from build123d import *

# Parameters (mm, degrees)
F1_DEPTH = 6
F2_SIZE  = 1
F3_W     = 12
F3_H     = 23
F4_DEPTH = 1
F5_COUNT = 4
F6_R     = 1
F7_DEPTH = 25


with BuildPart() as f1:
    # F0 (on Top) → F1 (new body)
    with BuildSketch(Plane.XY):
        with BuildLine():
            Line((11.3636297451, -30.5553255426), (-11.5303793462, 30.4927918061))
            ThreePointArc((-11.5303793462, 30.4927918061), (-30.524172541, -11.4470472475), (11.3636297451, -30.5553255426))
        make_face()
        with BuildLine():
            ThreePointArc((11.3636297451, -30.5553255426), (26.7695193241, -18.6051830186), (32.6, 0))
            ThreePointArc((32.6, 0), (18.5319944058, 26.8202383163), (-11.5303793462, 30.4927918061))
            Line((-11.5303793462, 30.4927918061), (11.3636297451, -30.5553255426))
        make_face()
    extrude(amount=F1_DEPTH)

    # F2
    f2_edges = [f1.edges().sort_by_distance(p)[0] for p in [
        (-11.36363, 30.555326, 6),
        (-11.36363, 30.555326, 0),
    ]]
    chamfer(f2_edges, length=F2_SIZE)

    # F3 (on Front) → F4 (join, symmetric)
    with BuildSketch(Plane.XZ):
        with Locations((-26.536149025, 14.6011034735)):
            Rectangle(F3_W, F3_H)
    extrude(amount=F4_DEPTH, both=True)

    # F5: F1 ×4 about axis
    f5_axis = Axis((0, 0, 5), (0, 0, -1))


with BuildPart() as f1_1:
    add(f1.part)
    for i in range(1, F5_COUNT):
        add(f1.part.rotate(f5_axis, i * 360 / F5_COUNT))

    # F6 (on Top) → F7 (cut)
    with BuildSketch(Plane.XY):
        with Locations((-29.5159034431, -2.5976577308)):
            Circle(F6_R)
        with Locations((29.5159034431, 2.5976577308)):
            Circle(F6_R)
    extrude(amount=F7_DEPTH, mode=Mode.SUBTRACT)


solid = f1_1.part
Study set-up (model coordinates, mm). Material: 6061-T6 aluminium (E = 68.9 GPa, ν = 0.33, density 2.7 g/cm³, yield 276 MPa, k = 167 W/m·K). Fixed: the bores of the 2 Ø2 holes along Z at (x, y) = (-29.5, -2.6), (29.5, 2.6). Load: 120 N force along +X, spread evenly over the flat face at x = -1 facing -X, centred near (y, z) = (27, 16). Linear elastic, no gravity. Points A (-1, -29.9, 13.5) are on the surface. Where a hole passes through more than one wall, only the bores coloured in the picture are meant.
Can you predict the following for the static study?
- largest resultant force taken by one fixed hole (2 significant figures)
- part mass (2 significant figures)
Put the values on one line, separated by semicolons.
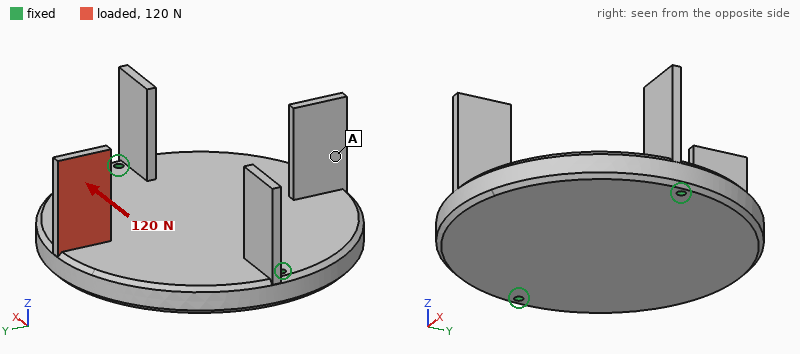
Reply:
90 N; 59 g
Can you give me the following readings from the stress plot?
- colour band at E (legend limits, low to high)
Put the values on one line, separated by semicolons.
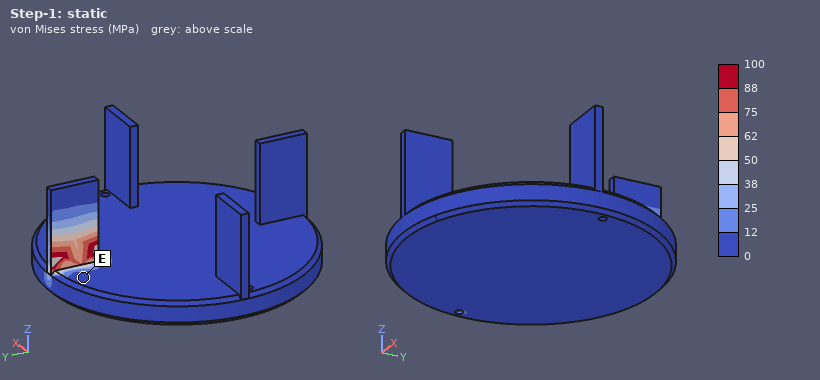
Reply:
0 to 12 MPa
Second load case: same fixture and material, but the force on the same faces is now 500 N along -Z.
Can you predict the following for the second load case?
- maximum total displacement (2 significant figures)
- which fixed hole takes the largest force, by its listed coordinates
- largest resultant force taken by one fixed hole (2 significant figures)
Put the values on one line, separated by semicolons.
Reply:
0.26 mm; (29.5, 2.6); 260 N
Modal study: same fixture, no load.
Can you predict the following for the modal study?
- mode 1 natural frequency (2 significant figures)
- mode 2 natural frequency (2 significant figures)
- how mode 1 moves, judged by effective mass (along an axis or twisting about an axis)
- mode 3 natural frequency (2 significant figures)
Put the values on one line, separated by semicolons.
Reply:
2500 Hz; 3700 Hz; twisting about X; 3800 Hz
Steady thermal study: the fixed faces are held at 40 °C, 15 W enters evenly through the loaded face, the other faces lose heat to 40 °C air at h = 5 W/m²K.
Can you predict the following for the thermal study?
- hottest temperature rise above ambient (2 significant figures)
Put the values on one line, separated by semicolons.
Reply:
56 K
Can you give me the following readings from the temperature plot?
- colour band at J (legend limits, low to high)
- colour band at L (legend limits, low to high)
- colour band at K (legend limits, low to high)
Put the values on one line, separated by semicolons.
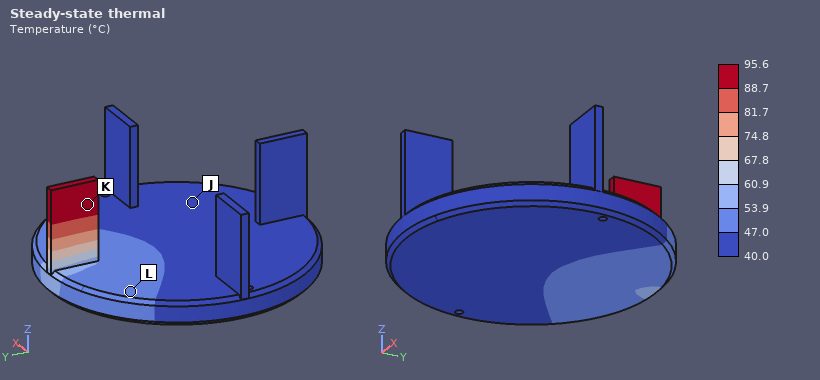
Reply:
40.0 to 47.0 °C; 47.0 to 53.9 °C; 88.7 to 95.6 °C
